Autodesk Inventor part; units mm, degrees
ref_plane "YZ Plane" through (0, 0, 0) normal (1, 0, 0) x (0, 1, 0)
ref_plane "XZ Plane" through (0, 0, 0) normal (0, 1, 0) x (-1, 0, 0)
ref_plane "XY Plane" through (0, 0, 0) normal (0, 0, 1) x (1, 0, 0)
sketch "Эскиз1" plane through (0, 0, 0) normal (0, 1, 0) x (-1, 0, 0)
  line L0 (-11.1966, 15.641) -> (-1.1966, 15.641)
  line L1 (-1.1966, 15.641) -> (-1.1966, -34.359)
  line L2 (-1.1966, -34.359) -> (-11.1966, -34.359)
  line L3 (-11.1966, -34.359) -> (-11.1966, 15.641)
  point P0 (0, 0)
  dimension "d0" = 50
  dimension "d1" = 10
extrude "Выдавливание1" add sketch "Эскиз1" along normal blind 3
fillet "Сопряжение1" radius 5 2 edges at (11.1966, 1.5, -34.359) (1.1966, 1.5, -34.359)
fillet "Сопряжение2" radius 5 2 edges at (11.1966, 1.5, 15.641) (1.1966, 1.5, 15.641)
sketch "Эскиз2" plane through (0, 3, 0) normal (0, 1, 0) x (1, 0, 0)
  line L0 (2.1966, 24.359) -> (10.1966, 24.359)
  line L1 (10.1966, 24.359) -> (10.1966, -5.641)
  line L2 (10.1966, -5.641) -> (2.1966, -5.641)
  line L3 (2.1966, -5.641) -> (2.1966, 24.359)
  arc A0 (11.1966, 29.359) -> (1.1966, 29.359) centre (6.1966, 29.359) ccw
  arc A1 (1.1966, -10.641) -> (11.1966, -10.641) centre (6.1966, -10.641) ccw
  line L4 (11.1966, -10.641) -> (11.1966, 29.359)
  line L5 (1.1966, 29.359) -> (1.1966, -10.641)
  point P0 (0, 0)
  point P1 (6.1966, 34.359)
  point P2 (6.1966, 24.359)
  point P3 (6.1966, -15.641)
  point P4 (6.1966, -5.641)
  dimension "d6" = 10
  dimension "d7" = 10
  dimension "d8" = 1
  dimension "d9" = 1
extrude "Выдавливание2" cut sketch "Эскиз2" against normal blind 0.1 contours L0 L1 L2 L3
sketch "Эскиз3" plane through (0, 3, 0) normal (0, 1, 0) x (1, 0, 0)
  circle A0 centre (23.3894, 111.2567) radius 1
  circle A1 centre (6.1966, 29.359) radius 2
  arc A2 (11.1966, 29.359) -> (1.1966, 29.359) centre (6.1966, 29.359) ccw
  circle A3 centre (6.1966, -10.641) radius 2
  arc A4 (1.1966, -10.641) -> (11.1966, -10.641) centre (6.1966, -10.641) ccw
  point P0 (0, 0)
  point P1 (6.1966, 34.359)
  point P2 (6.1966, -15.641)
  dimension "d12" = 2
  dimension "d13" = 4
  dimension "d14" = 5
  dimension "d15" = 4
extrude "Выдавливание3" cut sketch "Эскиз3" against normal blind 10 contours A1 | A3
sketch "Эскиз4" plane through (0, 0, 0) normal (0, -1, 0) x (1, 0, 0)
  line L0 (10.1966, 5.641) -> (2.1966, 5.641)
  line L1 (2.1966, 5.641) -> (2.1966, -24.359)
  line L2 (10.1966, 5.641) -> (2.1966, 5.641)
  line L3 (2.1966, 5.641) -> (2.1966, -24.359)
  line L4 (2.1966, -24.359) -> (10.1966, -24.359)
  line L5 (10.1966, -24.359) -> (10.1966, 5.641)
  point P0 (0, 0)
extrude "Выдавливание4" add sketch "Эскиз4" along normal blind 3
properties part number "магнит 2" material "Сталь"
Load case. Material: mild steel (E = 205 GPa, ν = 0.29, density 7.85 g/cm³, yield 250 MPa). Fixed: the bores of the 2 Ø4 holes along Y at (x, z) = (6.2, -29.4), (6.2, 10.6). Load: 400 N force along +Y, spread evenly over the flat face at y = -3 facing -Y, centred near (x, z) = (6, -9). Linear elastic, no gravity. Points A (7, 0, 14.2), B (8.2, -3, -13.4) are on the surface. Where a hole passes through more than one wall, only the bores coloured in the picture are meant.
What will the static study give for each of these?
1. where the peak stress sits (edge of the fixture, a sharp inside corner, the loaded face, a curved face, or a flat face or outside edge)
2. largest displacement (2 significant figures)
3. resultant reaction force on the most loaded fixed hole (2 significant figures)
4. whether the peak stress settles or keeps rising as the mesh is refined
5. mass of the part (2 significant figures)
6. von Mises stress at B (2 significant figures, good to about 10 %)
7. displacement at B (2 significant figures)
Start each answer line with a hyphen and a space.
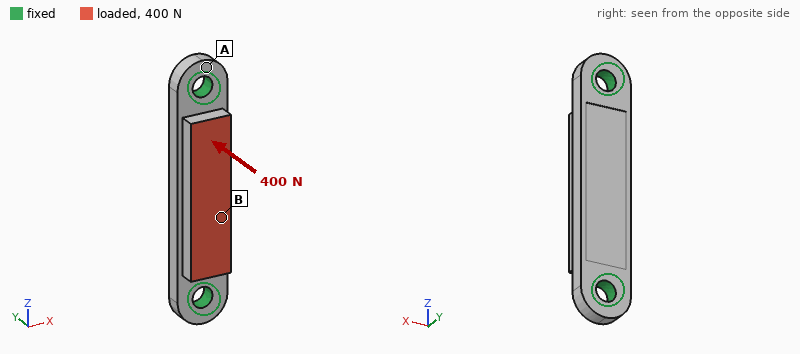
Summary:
- edge of the fixture
- 5.1 µm
- 290 N
- keeps rising
- 16 g
- 25 MPa
- 4.7 µm
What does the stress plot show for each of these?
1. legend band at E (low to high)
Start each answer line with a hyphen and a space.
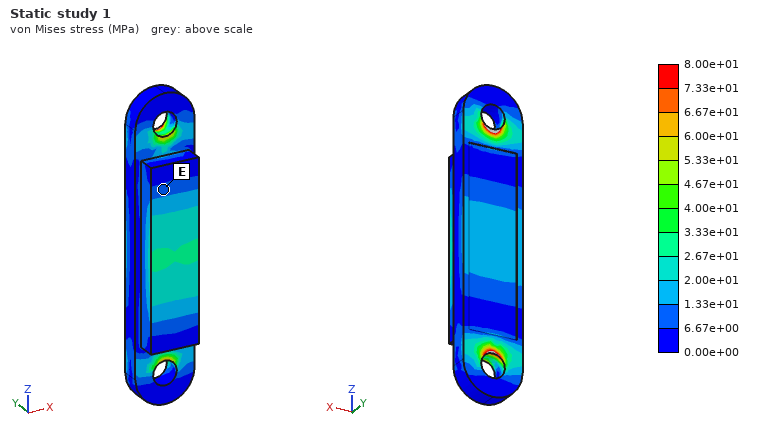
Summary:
- 6.67e+00 to 1.33e+01 MPa
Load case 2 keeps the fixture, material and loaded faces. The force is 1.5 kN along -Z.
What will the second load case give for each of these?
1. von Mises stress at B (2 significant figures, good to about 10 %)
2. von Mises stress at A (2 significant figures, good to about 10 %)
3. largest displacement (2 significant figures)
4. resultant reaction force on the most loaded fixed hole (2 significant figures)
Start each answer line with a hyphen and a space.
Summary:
- 11 MPa
- 5.2 MPa
- 1.9 µm
- 780 N
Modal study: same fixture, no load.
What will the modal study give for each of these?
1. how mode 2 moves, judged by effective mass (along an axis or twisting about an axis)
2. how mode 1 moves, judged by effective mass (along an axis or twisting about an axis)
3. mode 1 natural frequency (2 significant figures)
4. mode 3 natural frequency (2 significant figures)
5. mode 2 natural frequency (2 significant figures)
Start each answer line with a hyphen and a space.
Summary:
- along X
- along Y
- 14 kHz
- 24 kHz
- 18 kHz
